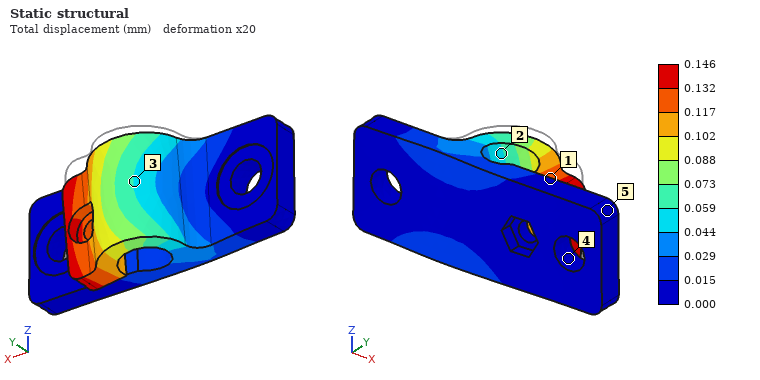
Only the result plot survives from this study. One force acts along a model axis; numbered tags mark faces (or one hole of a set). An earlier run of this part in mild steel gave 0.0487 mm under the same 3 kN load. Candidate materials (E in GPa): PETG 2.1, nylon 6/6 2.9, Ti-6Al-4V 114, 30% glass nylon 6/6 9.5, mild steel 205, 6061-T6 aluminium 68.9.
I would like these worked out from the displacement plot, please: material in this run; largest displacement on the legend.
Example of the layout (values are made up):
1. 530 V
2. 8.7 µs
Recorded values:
1. 6061-T6 aluminium
2. 0.146 mm
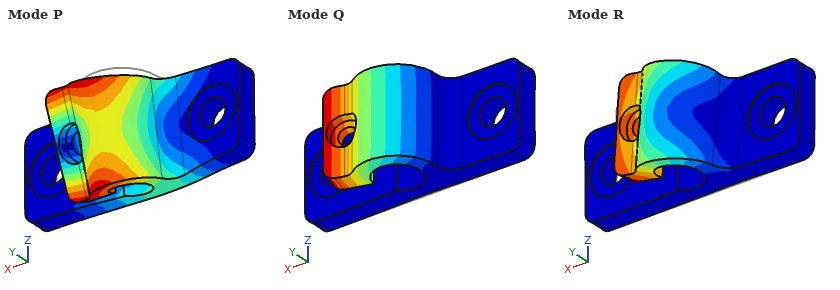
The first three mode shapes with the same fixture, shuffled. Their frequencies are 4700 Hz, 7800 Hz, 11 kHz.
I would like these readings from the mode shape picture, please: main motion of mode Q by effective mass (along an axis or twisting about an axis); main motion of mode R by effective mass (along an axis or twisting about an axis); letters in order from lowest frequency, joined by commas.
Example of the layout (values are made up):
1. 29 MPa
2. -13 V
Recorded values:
1. along Y
2. along Z
3. Q, R, P
